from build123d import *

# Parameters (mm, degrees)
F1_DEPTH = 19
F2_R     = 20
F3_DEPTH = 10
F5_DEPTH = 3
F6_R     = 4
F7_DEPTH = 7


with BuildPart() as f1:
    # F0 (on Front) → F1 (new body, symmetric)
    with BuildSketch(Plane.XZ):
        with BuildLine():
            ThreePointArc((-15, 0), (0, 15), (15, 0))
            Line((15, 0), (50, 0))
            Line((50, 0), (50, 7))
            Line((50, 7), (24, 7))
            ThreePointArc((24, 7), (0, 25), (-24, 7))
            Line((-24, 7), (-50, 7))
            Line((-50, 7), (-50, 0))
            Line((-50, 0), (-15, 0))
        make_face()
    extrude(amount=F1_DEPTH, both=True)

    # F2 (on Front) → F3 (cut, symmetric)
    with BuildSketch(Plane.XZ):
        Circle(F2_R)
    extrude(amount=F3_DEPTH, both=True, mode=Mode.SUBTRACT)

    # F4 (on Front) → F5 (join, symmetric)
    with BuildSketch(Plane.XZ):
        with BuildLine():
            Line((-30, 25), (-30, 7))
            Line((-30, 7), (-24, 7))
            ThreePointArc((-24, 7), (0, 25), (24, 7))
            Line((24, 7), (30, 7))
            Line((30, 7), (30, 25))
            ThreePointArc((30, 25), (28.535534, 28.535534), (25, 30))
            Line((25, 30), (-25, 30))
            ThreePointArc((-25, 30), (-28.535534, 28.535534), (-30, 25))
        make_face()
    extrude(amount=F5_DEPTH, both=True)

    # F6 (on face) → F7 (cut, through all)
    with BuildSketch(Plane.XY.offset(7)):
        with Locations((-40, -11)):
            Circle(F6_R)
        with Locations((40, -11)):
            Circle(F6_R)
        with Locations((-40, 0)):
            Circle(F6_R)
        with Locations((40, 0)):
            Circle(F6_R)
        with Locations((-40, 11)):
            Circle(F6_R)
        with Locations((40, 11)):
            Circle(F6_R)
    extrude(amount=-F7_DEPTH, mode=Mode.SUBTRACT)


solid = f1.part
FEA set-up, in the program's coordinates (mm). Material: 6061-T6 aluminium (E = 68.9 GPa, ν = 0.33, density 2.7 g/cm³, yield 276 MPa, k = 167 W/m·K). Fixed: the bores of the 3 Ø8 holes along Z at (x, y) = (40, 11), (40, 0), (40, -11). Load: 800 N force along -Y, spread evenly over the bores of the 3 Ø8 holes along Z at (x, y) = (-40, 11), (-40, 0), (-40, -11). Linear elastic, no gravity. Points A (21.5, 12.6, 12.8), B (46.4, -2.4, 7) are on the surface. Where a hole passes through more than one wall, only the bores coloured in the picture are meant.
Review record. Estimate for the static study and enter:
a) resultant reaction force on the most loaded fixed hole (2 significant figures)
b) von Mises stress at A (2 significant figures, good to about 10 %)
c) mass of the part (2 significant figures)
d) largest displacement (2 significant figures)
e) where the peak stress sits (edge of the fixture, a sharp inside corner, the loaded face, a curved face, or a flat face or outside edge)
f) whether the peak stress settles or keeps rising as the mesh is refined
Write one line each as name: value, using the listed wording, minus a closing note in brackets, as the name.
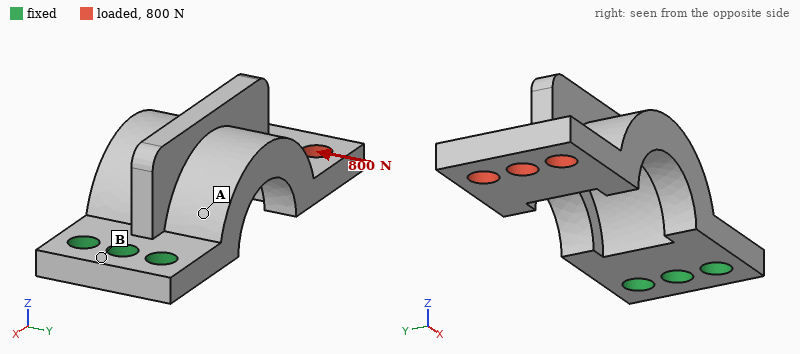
resultant reaction force on the most loaded fixed hole: 2.3 kN
von Mises stress at A: 53 MPa
mass of the part: 92 g
largest displacement: 0.40 mm
where the peak stress sits: a sharp inside corner
whether the peak stress settles or keeps rising as the mesh is refined: keeps rising
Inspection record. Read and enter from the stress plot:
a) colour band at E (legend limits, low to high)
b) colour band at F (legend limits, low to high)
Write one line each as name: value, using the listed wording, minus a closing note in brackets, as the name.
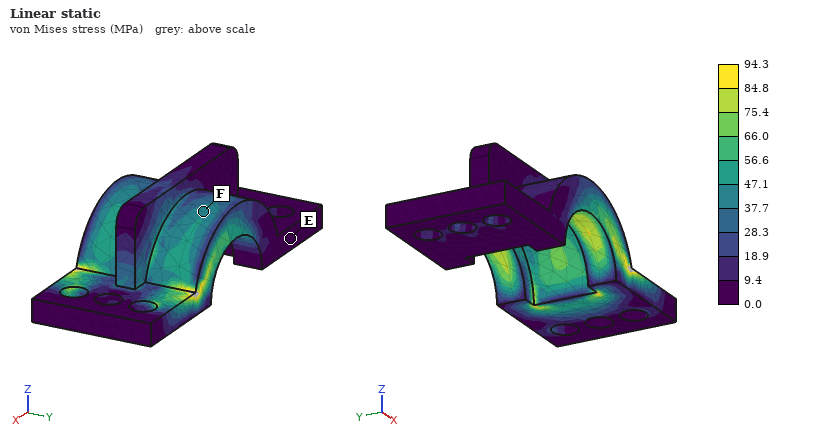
colour band at E: 0.0 to 9.4 MPa
colour band at F: 37.7 to 47.1 MPa
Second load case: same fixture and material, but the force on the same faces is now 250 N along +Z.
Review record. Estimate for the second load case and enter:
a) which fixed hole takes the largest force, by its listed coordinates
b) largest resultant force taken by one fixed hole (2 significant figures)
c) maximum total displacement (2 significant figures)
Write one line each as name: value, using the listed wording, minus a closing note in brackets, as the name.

which fixed hole takes the largest force, by its listed coordinates: (40, 0)
largest resultant force taken by one fixed hole: 310 N
maximum total displacement: 0.39 mm
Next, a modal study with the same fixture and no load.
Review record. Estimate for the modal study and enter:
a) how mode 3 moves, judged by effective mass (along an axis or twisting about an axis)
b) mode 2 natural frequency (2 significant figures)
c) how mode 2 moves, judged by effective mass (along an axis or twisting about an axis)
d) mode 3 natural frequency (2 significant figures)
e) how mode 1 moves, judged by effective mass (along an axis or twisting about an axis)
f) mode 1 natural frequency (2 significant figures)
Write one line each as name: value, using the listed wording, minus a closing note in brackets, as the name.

how mode 3 moves, judged by effective mass: along X
mode 2 natural frequency: 1600 Hz
how mode 2 moves, judged by effective mass: along Y
mode 3 natural frequency: 3600 Hz
how mode 1 moves, judged by effective mass: along Z
mode 1 natural frequency: 840 Hz
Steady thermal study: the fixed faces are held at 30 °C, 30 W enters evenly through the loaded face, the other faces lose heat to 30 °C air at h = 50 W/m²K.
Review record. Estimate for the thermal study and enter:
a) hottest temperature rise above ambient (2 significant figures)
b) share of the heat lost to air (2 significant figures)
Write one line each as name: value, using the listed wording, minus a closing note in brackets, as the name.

hottest temperature rise above ambient: 44 K
share of the heat lost to air: 38 %
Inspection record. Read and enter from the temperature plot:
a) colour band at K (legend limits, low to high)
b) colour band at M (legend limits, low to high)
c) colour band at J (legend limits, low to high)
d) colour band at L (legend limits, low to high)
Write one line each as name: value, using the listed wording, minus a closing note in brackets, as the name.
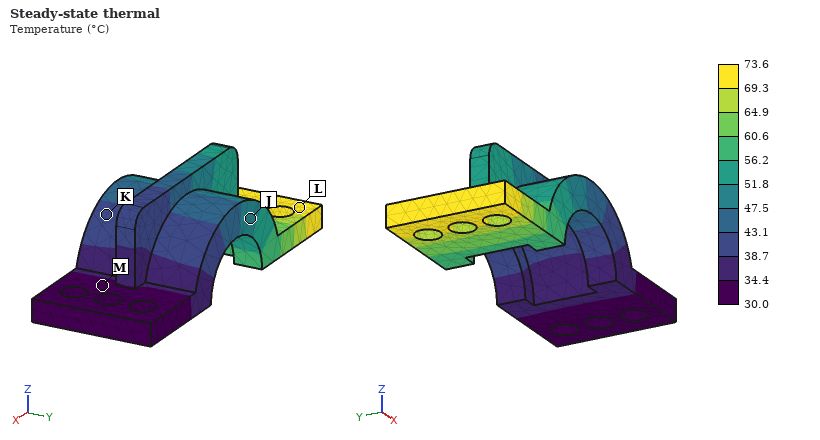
colour band at K: 38.7 to 43.1 °C
colour band at M: 30.0 to 34.4 °C
colour band at J: 47.5 to 51.8 °C
colour band at L: 69.3 to 73.6 °C
